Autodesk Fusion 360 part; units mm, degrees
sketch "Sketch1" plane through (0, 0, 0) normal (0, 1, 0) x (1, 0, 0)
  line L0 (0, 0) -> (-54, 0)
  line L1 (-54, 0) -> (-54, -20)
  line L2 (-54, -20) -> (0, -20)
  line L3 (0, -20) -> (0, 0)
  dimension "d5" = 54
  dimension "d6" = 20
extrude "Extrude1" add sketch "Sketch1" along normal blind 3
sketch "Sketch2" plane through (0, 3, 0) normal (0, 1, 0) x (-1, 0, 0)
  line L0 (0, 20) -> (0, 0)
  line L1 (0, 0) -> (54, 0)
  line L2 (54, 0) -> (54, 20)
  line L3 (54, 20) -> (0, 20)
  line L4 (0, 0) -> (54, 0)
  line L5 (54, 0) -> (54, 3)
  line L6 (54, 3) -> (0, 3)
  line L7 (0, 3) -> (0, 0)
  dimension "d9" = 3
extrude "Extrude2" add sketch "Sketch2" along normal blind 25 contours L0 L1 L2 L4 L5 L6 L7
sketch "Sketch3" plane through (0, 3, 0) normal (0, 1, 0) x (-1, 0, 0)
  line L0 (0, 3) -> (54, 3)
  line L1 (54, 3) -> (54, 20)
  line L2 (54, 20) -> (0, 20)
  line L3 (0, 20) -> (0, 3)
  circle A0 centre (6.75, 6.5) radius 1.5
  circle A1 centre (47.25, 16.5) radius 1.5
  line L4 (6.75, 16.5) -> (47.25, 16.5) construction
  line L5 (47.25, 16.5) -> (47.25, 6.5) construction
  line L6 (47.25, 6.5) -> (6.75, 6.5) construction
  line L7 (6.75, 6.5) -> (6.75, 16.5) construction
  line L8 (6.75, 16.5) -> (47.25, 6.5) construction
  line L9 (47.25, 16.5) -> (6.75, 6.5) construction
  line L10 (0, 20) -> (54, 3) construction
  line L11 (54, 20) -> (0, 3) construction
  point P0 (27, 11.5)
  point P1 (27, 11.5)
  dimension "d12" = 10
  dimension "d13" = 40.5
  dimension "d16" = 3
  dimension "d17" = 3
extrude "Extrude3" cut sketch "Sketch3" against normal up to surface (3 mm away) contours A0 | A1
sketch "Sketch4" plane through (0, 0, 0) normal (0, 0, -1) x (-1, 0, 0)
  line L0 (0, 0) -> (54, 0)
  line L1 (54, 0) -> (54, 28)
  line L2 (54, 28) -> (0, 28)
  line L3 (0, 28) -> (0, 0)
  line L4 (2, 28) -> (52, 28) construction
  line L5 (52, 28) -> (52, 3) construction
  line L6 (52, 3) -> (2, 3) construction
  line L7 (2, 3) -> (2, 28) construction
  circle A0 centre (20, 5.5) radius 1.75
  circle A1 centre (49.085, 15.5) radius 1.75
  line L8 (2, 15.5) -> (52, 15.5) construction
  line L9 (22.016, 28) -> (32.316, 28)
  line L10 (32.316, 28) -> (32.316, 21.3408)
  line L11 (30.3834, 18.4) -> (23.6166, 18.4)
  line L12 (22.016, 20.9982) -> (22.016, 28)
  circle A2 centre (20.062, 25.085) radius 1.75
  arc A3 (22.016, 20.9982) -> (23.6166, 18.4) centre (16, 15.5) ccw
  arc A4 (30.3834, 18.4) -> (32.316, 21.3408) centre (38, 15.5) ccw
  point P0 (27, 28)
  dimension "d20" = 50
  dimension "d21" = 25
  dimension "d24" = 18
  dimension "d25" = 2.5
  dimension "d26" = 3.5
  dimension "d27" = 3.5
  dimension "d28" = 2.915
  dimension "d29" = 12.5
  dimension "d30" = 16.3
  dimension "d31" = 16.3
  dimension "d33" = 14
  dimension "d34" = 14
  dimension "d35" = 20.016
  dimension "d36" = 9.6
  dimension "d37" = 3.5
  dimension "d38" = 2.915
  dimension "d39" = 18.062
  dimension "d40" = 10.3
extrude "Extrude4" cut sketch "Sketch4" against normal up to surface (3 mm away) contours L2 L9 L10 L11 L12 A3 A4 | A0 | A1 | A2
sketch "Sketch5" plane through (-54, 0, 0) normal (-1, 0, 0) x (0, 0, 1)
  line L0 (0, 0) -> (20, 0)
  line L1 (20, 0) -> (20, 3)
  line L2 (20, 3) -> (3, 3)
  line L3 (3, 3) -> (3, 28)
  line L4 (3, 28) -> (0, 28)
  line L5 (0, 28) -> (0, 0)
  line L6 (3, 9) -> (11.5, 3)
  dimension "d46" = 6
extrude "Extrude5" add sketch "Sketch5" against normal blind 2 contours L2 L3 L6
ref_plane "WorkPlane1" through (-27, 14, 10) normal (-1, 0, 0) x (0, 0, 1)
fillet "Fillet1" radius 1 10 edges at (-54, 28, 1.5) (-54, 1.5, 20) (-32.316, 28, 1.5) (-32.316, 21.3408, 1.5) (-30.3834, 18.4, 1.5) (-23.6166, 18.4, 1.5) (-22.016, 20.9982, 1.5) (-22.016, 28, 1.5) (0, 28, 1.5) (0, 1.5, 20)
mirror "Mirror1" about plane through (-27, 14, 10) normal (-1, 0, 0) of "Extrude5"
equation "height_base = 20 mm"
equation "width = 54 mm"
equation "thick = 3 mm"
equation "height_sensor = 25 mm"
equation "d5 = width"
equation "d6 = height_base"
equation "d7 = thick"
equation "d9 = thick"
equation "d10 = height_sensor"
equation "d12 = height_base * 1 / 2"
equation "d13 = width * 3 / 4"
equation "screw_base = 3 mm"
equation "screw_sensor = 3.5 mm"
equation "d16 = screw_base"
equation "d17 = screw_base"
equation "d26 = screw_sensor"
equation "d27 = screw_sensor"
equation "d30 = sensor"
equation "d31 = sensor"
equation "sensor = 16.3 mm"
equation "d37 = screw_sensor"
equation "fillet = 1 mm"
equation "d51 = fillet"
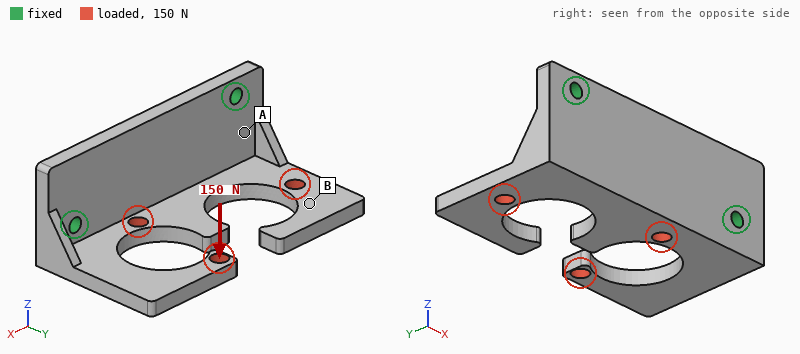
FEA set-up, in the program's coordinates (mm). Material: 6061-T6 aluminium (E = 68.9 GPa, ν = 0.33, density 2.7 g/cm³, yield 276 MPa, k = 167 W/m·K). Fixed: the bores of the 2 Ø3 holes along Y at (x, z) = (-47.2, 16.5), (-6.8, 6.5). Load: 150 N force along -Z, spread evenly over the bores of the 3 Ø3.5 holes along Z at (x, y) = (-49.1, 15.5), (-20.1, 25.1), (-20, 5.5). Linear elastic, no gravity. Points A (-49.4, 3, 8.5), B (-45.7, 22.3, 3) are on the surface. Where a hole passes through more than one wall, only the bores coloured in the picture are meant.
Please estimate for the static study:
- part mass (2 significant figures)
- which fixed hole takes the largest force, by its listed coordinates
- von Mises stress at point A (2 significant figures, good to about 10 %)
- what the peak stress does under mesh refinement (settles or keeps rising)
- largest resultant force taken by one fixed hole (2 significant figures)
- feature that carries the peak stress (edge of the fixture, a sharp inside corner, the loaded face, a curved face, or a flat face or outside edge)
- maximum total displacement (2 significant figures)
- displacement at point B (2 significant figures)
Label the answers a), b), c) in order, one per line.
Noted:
a) 15 g
b) (-47.2, 16.5)
c) 19 MPa
d) keeps rising
e) 89 N
f) edge of the fixture
g) 0.37 mm
h) 0.084 mm
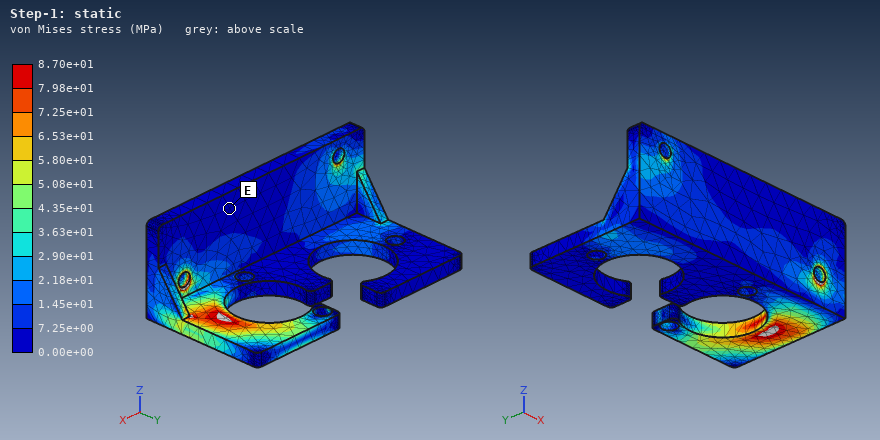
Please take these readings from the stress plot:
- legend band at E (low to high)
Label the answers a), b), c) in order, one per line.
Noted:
a) 0.00e+00 to 7.25e+00 MPa
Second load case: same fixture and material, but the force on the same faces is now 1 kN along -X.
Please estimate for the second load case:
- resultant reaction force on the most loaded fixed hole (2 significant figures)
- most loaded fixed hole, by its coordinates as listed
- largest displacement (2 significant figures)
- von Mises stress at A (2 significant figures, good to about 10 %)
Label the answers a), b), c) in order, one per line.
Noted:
a) 690 N
b) (-6.8, 6.5)
c) 0.25 mm
d) 46 MPa
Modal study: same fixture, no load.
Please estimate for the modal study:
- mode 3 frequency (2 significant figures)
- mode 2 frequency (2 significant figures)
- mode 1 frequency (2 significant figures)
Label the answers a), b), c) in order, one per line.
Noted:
a) 4600 Hz
b) 2800 Hz
c) 2100 Hz
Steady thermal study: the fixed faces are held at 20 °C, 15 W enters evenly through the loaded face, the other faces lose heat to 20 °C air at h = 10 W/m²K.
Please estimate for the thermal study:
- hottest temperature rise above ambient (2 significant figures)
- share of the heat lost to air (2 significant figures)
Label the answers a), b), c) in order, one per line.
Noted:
a) 61 K
b) 3.5 %
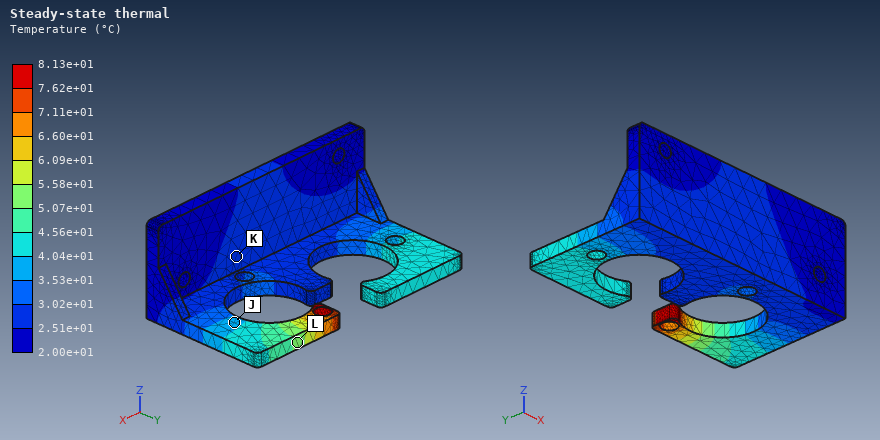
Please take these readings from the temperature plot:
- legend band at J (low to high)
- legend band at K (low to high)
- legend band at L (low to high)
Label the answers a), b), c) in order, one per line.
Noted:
a) 3.53e+01 to 4.04e+01 °C
b) 2.51e+01 to 3.02e+01 °C
c) 5.07e+01 to 5.58e+01 °C
